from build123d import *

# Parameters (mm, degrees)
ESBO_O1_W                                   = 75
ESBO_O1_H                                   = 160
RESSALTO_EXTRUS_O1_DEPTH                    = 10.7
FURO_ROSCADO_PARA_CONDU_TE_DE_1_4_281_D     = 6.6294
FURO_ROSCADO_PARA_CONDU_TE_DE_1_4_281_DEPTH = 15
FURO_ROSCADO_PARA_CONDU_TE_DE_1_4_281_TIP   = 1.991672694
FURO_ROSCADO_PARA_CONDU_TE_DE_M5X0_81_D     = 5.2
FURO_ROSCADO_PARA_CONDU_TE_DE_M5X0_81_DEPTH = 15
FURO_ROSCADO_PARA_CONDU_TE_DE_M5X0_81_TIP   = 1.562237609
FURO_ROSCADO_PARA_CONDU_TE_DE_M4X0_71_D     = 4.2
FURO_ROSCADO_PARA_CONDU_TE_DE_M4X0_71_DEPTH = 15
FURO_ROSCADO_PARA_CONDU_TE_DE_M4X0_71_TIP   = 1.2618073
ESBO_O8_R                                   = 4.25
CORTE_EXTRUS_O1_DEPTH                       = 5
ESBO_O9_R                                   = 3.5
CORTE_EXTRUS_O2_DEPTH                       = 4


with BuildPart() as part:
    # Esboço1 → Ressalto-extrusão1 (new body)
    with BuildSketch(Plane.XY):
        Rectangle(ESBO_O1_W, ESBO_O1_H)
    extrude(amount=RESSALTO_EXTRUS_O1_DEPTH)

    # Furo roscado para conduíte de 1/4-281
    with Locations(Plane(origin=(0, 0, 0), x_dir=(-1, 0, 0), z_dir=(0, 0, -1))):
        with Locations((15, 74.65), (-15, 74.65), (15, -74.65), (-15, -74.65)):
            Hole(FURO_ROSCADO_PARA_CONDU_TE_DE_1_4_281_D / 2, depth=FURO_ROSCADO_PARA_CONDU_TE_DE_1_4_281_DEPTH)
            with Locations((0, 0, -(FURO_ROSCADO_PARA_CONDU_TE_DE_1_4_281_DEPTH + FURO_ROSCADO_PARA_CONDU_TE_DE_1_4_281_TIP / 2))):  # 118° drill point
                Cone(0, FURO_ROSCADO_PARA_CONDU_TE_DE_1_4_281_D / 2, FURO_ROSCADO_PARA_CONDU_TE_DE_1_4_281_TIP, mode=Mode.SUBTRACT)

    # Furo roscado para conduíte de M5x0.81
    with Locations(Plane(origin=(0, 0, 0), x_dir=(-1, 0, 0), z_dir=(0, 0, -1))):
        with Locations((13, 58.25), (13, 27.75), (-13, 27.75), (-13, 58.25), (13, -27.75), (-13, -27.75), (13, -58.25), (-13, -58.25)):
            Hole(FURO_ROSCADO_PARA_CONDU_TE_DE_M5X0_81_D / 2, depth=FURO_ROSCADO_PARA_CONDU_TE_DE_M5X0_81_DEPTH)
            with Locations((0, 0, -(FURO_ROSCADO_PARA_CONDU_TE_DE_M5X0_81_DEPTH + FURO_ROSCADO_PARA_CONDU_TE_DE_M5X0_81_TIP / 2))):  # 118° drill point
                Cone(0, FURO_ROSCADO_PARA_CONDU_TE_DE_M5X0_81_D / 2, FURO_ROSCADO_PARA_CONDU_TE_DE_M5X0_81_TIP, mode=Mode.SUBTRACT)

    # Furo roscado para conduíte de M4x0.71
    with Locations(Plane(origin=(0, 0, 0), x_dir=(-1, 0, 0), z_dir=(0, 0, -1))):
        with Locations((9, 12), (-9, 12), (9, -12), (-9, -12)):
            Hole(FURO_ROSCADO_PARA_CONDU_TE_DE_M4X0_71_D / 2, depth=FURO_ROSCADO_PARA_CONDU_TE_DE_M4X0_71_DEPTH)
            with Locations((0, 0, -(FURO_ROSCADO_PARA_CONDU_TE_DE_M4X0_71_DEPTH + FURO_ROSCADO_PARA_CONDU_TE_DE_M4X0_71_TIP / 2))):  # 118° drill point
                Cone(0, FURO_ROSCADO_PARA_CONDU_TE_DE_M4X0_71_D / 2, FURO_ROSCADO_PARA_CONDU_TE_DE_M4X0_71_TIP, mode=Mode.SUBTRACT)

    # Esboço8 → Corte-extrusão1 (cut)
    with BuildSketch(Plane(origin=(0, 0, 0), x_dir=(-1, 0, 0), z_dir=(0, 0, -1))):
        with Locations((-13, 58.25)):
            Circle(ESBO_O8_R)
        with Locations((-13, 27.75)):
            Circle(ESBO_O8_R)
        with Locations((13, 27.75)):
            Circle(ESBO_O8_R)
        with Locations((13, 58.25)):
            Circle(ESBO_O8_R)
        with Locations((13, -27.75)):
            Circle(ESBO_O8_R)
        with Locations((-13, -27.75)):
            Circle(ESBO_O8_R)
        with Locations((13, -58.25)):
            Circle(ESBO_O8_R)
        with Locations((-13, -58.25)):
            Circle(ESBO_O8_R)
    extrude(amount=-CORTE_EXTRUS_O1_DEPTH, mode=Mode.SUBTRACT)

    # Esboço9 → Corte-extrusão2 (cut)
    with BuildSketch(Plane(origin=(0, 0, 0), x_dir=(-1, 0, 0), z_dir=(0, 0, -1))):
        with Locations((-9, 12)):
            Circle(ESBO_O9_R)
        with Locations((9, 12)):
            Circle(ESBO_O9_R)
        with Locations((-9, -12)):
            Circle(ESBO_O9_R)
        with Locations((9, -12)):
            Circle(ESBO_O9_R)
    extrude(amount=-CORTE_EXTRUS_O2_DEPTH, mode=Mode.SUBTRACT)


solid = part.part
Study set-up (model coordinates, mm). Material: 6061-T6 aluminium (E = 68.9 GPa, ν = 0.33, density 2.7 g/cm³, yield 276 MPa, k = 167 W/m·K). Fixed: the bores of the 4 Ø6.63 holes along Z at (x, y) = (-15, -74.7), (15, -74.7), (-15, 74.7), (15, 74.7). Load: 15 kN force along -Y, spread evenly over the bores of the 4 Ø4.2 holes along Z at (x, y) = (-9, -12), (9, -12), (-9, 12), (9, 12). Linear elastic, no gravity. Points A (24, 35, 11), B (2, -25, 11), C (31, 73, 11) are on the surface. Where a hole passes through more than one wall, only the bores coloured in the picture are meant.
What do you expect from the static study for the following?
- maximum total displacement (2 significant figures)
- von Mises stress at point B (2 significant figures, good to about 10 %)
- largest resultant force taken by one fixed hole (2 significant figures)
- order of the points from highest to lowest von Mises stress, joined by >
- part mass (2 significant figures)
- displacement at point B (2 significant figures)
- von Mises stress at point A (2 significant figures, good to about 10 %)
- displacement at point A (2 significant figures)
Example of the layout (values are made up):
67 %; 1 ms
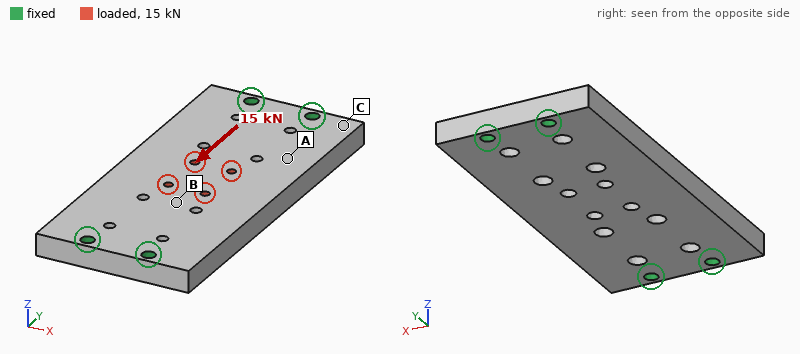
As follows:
20 µm; 23 MPa; 3.8 kN; B > A > C; 330 g; 13 µm; 13 MPa; 9.6 µm
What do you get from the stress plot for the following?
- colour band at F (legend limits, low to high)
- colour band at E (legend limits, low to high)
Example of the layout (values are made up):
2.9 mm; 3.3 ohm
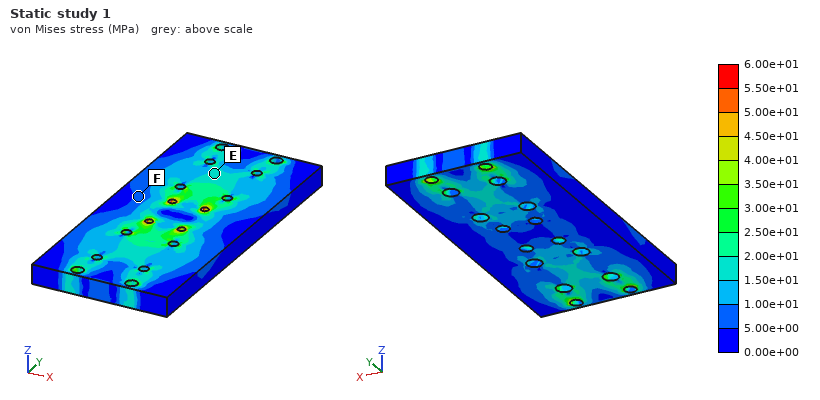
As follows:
5.00e+00 to 1.00e+01 MPa; 1.50e+01 to 2.00e+01 MPa
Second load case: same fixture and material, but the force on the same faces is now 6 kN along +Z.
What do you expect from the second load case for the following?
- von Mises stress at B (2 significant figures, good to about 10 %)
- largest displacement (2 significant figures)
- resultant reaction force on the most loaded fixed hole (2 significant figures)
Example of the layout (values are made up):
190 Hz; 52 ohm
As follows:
32 MPa; 0.23 mm; 1.5 kN
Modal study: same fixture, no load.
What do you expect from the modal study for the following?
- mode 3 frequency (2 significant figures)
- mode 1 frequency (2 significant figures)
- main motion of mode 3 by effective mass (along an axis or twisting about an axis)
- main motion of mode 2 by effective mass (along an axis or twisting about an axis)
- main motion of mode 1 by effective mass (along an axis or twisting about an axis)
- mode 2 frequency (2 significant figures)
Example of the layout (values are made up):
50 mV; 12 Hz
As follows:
5800 Hz; 2200 Hz; twisting about X; twisting about Y; along Z; 3200 Hz
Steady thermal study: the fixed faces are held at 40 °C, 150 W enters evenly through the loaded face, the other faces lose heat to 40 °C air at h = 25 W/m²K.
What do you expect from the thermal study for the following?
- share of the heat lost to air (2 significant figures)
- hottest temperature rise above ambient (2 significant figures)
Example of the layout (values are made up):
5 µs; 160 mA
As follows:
10 %; 47 K
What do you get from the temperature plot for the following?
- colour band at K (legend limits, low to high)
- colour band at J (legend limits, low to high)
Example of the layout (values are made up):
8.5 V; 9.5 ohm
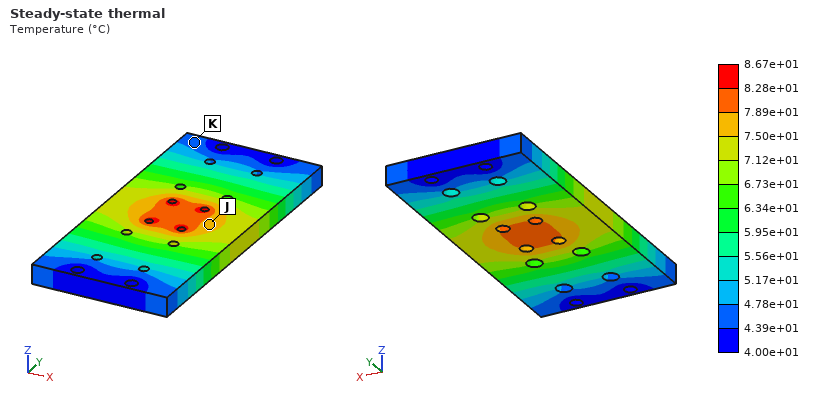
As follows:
4.39e+01 to 4.78e+01 °C; 7.50e+01 to 7.89e+01 °C
